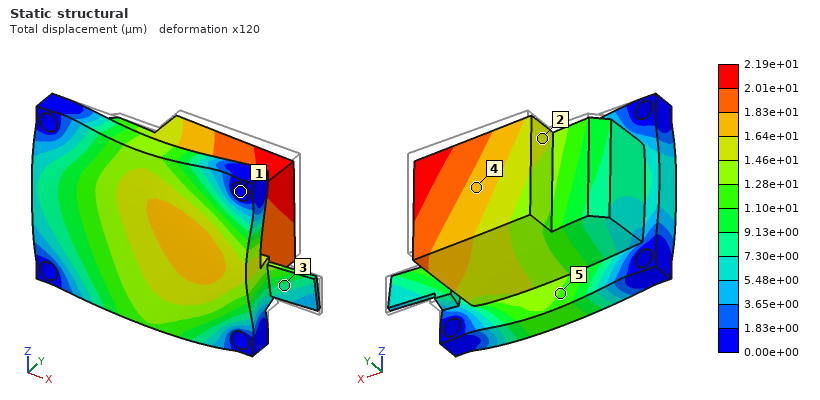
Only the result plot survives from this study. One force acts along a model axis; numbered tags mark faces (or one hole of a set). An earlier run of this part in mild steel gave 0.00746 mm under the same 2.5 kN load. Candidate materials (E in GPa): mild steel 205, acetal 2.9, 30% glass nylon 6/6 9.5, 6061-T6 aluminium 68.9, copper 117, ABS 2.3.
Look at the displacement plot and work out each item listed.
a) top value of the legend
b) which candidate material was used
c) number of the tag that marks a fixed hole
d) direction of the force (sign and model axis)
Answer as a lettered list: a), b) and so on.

a) 2.19e+01 µm
b) 6061-T6 aluminium
c) 1
d) -Y
